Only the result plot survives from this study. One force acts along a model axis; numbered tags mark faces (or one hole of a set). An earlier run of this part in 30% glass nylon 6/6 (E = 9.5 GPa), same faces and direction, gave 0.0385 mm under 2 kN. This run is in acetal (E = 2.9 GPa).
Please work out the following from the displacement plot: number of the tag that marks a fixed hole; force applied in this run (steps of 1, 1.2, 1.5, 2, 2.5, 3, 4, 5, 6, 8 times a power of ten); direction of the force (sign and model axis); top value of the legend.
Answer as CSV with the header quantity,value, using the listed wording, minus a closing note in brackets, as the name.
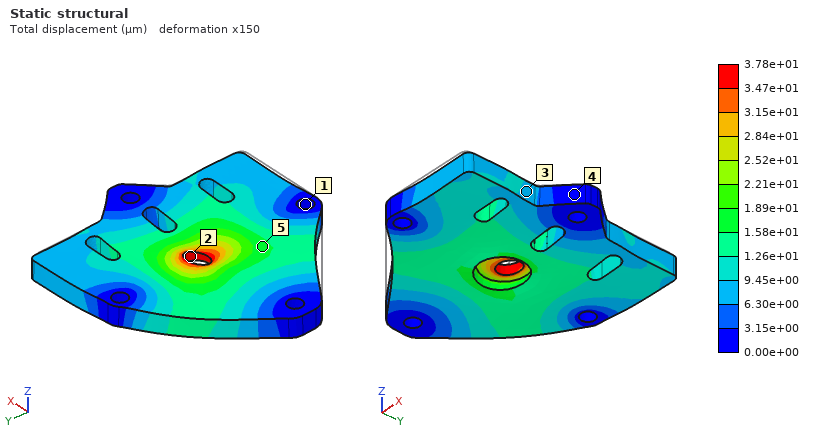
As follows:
quantity,value
number of the tag that marks a fixed hole,1
force applied in this run,600 N
direction of the force,+Y
top value of the legend,3.78e+01 µm
